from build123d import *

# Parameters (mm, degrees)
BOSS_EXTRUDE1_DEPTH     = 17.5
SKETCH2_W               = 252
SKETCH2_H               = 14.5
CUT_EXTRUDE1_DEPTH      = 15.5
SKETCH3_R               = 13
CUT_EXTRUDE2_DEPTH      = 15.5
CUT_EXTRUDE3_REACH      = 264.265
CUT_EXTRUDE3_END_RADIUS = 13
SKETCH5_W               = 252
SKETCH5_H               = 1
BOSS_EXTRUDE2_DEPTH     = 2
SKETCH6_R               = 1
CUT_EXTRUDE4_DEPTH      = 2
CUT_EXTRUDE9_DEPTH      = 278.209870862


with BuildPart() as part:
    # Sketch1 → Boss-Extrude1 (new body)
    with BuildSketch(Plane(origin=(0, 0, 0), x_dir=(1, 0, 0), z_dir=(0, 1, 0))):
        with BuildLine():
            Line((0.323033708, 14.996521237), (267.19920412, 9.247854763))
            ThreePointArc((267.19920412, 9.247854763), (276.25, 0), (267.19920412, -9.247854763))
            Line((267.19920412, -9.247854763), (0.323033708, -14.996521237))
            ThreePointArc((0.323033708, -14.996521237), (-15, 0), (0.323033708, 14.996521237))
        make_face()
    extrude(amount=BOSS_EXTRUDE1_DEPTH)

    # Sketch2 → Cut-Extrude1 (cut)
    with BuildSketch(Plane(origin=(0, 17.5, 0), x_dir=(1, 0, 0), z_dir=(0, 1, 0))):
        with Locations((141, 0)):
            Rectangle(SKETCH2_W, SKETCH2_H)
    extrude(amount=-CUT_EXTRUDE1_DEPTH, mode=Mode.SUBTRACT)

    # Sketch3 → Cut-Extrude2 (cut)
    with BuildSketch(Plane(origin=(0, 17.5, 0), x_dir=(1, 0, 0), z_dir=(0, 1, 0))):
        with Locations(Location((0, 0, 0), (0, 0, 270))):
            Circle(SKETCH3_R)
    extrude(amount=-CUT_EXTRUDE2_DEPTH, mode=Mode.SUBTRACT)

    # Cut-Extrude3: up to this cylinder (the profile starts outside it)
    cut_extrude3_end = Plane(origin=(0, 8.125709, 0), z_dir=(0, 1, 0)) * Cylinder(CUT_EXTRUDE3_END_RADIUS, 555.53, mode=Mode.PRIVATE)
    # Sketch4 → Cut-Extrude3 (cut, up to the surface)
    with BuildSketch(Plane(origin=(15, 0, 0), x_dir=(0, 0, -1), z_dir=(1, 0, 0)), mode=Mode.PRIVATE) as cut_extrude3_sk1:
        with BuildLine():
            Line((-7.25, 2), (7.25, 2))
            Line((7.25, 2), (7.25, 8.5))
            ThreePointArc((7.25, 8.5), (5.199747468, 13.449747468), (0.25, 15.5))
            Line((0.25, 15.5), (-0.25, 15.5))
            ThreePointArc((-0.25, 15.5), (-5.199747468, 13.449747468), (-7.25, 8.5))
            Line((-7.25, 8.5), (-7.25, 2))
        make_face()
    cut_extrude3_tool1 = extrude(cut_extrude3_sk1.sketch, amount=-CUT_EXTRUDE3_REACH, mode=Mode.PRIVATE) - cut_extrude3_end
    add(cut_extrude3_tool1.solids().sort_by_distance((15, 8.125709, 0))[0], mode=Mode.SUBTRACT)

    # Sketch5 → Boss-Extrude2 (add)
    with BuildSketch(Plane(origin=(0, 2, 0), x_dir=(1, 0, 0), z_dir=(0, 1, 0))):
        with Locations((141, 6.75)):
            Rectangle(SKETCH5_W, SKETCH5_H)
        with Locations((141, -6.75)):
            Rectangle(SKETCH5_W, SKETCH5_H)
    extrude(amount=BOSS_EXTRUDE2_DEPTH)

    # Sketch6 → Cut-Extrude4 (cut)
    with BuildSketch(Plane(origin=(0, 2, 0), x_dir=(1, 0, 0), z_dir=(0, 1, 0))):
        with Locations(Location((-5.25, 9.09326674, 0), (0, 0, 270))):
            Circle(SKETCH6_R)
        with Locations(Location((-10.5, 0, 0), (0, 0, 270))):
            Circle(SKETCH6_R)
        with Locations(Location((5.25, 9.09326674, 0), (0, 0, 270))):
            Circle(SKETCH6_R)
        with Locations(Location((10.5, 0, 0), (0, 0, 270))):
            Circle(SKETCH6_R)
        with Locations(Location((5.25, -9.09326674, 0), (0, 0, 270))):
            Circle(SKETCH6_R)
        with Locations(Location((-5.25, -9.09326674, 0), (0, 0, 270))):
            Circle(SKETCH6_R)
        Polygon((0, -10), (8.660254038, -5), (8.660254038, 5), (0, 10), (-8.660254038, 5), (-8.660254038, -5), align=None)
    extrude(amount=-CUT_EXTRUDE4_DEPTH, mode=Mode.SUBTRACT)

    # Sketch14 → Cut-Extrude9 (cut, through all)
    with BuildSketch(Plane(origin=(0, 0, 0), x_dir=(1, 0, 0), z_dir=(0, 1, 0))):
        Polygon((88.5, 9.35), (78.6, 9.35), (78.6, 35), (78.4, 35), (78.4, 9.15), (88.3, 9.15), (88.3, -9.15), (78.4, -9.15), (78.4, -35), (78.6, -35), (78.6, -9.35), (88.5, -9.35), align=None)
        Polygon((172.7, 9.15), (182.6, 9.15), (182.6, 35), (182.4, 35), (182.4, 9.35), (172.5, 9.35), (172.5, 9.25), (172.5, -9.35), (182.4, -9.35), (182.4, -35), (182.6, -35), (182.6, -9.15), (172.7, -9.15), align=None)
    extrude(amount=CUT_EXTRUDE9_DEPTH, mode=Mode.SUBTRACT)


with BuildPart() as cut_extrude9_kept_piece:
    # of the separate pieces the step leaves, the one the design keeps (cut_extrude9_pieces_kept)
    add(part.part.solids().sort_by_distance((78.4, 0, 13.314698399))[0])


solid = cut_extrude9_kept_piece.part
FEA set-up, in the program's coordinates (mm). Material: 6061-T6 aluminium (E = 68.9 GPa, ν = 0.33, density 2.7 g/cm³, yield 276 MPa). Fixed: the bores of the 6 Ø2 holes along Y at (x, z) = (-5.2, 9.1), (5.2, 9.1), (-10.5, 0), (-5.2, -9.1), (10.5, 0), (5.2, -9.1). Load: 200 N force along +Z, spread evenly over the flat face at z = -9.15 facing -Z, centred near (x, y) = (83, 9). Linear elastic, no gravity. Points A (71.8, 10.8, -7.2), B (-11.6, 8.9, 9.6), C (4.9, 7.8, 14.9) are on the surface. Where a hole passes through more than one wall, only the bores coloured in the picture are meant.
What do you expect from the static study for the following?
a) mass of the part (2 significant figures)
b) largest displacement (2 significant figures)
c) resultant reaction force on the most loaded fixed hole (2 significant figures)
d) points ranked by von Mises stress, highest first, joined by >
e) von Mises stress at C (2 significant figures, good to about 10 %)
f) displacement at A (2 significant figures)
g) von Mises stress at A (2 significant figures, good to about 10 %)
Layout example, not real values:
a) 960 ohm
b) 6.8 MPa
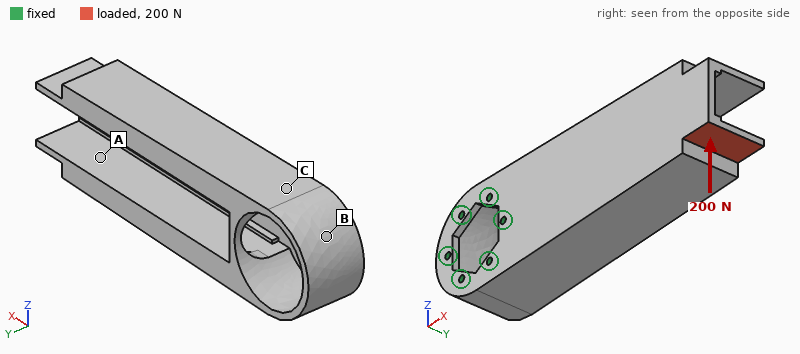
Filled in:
a) 62 g
b) 0.15 mm
c) 470 N
d) A > C > B
e) 9.8 MPa
f) 0.073 mm
g) 14 MPa
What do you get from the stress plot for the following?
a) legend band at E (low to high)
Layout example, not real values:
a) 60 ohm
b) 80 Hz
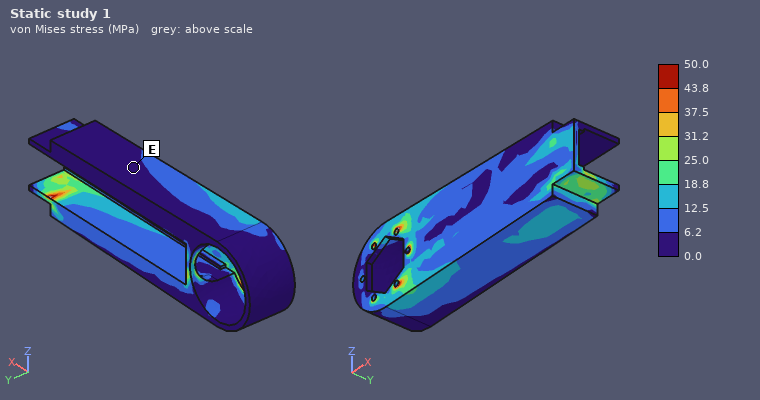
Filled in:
a) 0.0 to 6.2 MPa
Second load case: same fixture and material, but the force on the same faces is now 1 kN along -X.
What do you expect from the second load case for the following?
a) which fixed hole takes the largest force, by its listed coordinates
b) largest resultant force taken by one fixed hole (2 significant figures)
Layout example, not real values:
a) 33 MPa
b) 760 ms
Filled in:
a) (5.2, -9.1)
b) 560 N
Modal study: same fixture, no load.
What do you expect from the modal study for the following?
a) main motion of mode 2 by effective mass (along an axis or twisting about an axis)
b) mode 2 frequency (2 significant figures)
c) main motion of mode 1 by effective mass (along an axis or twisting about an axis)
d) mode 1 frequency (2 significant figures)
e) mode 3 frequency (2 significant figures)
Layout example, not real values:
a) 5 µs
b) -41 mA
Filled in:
a) along Z
b) 1900 Hz
c) along Y
d) 1100 Hz
e) 2900 Hz
